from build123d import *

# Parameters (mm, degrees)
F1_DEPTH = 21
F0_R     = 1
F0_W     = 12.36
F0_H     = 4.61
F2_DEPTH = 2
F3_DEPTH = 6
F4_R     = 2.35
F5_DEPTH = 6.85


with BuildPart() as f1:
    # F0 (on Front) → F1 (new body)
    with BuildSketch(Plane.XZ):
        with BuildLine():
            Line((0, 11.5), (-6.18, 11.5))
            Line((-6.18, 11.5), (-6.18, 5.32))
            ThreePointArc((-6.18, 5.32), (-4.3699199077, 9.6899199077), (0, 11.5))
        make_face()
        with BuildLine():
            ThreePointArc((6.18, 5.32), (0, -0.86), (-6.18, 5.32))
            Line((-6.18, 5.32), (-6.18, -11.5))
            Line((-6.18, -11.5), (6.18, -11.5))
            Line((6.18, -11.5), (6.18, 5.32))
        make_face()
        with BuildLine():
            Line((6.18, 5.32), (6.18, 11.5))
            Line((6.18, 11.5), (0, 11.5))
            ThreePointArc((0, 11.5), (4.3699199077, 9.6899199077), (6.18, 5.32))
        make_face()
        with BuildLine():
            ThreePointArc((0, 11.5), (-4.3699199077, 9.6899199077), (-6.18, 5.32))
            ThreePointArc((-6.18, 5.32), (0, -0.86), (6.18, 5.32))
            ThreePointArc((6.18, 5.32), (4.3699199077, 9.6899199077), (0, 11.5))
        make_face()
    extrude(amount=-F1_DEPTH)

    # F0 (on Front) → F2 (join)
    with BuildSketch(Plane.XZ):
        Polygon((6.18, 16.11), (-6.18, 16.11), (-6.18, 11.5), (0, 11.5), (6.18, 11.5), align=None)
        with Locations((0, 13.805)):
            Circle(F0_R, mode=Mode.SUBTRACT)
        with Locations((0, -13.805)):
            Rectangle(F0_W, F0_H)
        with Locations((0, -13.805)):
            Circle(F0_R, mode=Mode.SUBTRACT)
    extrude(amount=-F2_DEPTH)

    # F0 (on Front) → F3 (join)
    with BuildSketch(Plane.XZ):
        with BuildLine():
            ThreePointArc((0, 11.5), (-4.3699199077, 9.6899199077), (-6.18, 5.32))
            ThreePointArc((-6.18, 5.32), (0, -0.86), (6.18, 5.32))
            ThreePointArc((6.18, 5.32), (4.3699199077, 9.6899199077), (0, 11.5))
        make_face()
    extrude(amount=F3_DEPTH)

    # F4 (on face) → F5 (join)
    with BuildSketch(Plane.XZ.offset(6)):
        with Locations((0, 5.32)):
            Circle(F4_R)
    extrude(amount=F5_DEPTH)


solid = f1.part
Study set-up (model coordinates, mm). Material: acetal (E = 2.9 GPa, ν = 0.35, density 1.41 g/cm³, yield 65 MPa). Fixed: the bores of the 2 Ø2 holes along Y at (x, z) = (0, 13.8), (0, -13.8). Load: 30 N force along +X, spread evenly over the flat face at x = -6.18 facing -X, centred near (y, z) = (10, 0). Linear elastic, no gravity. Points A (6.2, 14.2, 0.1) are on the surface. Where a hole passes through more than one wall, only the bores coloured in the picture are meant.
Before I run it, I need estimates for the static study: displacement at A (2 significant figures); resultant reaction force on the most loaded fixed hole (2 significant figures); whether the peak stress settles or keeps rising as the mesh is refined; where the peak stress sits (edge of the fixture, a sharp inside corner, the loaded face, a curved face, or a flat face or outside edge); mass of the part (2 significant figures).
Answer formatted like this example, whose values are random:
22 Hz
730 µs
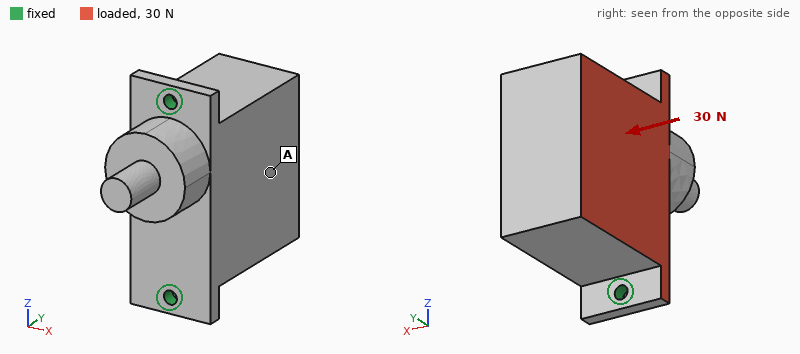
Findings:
0.17 mm
15 N
keeps rising
edge of the fixture
9.9 g
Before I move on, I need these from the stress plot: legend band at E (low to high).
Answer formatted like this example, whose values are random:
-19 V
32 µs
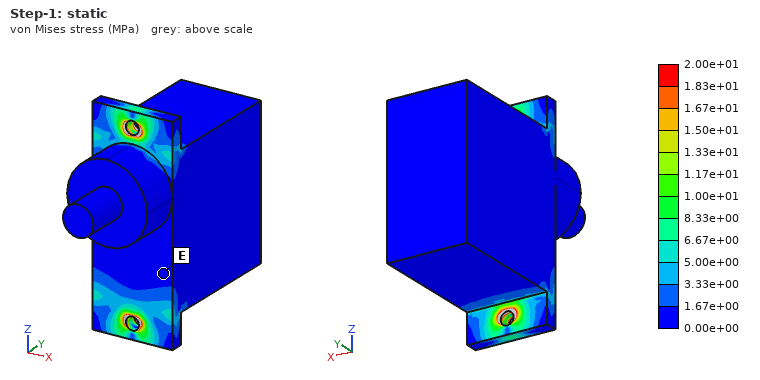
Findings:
0.00e+00 to 1.67e+00 MPa
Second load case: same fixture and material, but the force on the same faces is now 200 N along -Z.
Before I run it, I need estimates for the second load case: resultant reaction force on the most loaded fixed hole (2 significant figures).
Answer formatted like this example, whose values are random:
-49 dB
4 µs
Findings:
130 N
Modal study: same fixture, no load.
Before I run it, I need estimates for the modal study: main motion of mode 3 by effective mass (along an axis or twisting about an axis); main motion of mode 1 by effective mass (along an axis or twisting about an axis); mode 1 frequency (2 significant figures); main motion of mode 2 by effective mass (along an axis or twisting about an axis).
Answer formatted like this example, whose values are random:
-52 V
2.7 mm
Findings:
along Y
along X
690 Hz
along Z
